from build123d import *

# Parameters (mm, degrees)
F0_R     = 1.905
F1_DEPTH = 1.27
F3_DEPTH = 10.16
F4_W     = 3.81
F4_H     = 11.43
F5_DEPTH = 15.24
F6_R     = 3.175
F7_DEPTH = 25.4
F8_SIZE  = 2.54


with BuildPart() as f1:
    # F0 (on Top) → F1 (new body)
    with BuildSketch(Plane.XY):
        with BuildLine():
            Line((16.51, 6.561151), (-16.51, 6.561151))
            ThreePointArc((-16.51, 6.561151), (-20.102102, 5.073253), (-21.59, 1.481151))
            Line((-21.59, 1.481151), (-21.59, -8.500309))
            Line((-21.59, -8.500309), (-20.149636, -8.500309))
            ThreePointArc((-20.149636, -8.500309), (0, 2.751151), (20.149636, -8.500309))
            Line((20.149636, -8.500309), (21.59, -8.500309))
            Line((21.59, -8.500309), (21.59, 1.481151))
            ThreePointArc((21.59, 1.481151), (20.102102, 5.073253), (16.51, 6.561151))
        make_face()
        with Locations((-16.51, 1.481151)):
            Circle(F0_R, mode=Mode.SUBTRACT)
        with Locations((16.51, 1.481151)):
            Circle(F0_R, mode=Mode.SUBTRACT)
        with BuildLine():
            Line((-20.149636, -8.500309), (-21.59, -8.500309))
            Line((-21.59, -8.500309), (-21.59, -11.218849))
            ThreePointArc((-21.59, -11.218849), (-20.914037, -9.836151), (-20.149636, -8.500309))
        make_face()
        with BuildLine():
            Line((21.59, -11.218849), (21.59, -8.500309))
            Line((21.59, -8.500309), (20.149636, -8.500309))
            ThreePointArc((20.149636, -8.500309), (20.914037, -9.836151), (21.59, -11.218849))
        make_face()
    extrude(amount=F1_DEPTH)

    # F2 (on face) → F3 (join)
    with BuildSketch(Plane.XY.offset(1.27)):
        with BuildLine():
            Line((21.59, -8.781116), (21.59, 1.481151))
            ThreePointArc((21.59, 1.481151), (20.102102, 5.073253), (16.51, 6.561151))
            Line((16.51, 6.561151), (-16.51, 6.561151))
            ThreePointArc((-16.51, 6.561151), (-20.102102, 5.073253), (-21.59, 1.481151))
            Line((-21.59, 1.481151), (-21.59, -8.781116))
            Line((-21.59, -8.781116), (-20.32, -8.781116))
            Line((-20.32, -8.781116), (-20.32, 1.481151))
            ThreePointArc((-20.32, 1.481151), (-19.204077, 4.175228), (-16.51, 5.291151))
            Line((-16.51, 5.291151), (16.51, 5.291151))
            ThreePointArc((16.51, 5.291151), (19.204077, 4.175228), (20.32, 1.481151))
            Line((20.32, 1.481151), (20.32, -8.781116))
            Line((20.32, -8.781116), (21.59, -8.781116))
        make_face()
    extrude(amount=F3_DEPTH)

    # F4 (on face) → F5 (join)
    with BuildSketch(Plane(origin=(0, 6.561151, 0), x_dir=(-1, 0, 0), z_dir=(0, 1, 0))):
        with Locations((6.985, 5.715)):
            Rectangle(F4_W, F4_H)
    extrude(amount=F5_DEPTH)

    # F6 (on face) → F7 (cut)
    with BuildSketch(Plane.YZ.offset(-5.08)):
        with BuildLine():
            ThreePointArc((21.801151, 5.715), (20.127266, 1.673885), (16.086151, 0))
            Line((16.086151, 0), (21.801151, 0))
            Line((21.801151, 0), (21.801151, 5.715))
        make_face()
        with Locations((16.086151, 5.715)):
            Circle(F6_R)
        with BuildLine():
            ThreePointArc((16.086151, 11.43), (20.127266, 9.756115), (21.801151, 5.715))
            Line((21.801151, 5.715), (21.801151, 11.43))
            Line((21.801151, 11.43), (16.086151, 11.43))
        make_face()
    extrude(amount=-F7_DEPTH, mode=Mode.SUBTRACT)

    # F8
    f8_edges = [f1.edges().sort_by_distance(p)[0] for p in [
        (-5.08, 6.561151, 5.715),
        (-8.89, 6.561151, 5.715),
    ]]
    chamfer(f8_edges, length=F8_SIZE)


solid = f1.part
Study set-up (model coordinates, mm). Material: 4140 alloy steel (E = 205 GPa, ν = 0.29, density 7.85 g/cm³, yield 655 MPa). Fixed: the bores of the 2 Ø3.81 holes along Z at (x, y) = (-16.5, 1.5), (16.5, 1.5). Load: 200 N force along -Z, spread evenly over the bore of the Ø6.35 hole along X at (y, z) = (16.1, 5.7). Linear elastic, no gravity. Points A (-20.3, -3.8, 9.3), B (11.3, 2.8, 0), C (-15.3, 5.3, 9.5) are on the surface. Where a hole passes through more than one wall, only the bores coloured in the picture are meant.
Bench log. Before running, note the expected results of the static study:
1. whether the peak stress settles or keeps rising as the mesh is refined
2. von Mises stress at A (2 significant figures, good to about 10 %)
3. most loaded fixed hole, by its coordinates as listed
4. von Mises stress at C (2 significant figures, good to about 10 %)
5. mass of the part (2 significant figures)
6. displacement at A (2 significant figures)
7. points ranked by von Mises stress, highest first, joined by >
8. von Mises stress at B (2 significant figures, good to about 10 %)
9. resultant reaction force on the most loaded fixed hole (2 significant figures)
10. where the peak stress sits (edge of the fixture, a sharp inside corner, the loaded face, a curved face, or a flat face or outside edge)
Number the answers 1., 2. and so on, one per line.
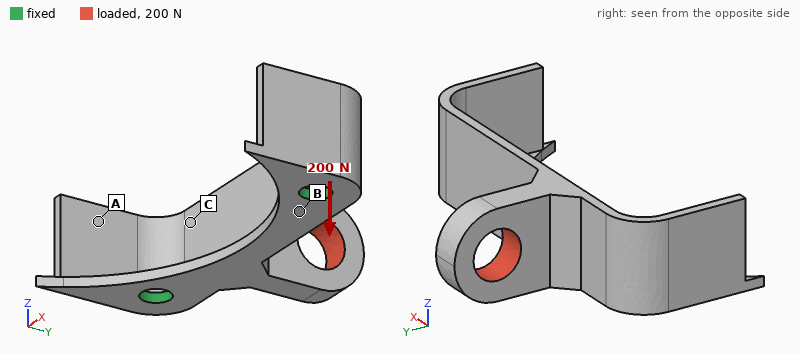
1. keeps rising
2. 35 MPa
3. (-16.5, 1.5)
4. 140 MPa
5. 14 g
6. 0.046 mm
7. C > B > A
8. 96 MPa
9. 150 N
10. edge of the fixture
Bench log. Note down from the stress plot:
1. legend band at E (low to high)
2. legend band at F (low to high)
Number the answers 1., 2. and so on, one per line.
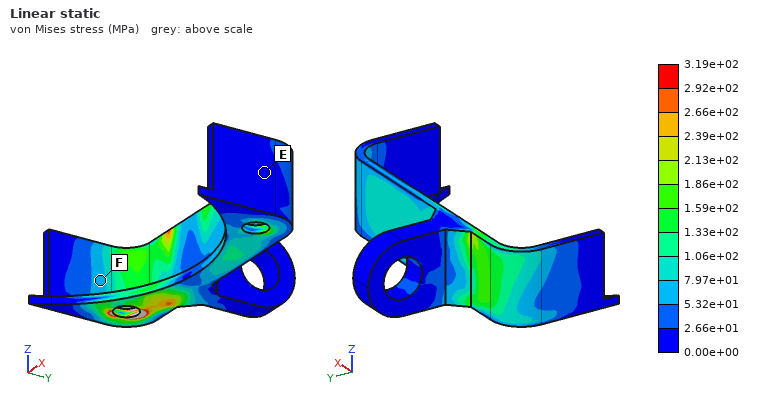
1. 0.00e+00 to 2.66e+01 MPa
2. 5.32e+01 to 7.97e+01 MPa
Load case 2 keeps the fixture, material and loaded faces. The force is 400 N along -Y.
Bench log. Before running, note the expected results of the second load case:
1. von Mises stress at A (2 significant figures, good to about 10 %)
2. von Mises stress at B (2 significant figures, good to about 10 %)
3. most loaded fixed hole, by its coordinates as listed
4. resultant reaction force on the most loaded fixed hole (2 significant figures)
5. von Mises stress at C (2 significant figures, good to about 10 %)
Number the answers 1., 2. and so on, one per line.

1. 31 MPa
2. 90 MPa
3. (-16.5, 1.5)
4. 350 N
5. 130 MPa
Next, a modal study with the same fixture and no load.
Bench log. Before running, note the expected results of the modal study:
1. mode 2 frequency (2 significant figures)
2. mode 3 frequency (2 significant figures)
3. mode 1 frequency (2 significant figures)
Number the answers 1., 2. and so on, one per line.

1. 8300 Hz
2. 9100 Hz
3. 3000 Hz
